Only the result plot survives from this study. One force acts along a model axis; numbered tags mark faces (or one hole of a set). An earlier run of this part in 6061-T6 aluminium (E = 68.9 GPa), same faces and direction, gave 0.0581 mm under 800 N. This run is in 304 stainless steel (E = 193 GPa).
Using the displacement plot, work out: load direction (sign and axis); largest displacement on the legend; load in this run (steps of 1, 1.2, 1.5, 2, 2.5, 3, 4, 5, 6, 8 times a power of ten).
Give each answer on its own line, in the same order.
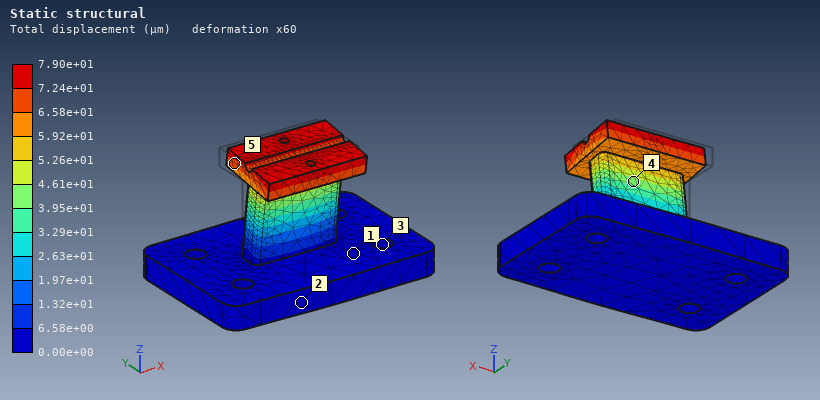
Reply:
-Y
7.90e+01 µm
3 kN
